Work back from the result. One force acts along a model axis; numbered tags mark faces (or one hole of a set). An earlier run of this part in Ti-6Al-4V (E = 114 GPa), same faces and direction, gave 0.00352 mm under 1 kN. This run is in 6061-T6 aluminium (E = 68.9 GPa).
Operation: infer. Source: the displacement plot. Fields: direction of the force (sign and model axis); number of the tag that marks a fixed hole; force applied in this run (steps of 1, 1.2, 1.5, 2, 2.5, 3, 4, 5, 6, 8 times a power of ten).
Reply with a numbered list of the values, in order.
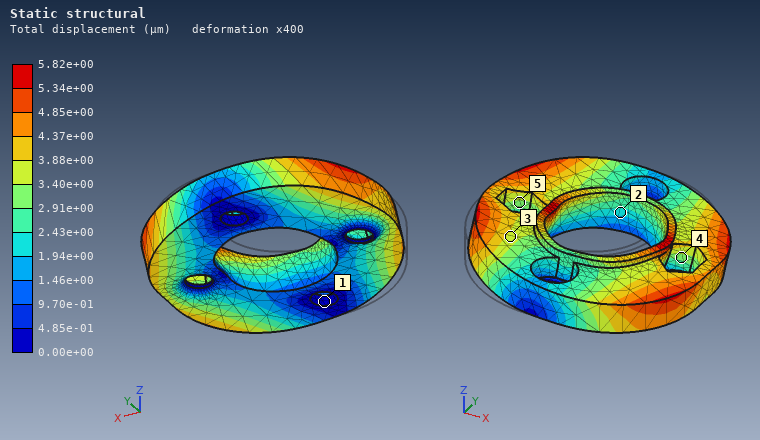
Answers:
1. +X
2. 1
3. 1 kN
